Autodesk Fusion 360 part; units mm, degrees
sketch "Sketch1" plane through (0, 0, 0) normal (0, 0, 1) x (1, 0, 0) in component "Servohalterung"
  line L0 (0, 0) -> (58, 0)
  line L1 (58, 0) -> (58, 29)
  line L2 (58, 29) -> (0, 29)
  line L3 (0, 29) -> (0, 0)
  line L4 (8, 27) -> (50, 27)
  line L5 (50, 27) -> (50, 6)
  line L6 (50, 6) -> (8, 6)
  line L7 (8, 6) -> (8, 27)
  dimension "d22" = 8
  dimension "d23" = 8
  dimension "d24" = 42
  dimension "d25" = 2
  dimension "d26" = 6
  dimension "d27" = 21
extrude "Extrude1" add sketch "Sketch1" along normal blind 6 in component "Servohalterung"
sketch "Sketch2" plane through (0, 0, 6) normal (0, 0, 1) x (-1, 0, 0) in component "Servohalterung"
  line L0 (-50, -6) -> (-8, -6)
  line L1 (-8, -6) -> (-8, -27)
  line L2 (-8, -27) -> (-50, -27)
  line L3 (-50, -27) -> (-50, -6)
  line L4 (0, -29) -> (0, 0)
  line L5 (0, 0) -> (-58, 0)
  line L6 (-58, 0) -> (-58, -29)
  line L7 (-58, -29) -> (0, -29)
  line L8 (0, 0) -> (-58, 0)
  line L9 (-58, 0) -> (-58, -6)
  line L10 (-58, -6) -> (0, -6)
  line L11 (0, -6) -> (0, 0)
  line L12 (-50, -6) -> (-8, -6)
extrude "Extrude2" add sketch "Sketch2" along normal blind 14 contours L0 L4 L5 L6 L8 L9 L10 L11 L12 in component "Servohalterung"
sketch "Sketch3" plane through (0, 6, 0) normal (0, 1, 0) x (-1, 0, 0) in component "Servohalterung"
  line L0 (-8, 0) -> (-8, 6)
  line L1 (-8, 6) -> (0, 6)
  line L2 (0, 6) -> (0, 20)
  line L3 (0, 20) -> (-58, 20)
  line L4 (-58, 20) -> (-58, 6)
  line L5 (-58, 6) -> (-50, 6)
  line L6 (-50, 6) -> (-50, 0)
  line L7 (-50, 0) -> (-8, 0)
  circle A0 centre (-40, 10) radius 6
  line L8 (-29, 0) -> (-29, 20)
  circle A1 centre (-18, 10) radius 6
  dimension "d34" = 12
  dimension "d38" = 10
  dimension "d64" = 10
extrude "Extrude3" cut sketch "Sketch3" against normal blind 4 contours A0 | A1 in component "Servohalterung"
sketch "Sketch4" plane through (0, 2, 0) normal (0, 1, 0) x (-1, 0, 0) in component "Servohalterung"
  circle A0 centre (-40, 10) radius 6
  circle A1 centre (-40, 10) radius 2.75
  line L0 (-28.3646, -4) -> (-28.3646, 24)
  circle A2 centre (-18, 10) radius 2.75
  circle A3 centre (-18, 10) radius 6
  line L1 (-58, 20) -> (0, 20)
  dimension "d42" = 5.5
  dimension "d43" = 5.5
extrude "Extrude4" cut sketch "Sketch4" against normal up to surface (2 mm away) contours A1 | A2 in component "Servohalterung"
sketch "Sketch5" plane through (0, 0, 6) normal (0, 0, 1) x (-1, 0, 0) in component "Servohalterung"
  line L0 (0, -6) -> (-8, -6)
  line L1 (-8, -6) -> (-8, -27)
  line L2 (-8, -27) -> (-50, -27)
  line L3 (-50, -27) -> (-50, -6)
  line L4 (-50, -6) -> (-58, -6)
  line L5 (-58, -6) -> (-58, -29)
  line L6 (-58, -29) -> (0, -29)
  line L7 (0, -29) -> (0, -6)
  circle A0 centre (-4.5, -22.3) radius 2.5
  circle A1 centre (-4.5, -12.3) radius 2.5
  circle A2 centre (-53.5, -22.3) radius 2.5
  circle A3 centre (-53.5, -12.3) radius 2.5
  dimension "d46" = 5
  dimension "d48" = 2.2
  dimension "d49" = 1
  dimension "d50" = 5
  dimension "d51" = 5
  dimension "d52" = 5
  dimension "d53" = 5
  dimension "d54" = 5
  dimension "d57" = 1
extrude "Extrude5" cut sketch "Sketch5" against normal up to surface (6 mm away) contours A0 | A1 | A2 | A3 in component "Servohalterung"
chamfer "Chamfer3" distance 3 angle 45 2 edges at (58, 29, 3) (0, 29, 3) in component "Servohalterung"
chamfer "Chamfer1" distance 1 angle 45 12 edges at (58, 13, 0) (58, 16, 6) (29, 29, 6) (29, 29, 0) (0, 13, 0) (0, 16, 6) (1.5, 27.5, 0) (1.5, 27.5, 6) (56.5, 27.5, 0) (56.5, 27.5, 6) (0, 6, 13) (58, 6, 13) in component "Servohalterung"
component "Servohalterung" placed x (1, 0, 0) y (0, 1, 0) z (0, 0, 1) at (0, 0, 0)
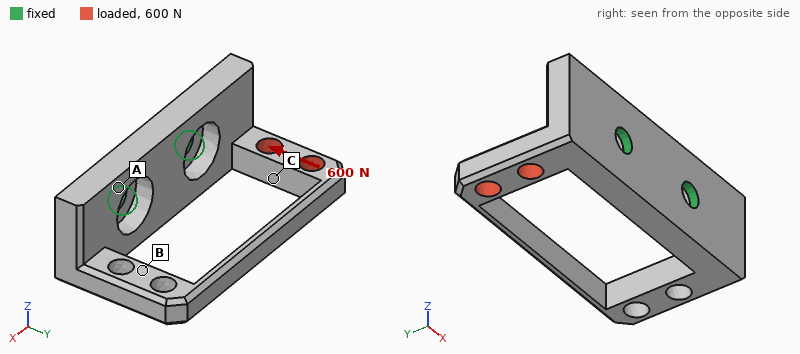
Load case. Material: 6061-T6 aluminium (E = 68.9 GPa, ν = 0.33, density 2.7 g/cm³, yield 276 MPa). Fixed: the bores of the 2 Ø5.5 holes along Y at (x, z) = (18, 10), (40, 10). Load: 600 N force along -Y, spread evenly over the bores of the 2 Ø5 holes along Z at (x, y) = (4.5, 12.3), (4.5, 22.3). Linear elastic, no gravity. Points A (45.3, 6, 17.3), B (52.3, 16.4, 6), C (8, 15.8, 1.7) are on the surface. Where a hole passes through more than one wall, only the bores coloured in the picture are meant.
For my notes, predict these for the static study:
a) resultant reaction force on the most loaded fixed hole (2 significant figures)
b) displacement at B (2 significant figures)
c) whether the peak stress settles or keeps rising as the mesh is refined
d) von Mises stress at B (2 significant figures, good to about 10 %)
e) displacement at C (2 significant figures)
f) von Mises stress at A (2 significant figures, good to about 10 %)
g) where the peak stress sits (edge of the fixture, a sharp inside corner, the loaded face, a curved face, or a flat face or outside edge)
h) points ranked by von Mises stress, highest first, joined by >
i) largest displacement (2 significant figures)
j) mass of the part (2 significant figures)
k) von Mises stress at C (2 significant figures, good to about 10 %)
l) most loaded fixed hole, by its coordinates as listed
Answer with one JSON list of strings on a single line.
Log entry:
["900 N", "0.035 mm", "keeps rising", "12 MPa", "0.093 mm", "22 MPa", "edge of the fixture", "C > A > B", "0.14 mm", "22 g", "42 MPa", "(18, 10)"]
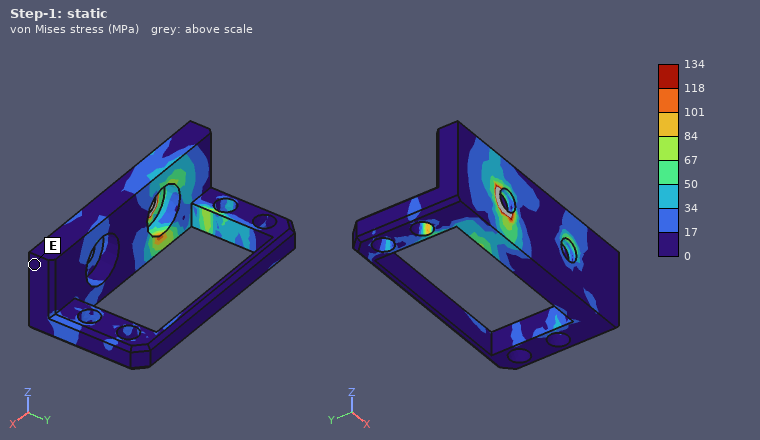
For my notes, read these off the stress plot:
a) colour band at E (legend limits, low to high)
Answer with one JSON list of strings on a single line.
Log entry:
["0 to 17 MPa"]
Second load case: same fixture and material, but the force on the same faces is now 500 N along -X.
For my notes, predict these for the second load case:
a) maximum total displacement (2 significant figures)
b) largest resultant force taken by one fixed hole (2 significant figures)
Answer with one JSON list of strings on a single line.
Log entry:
["0.15 mm", "410 N"]
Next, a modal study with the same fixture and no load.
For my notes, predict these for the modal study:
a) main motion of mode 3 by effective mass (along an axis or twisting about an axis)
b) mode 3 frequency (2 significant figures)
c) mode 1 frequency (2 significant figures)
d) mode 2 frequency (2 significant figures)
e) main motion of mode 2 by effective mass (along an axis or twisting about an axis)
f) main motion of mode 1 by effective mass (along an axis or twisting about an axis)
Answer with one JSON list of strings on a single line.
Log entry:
["twisting about Y", "4700 Hz", "3000 Hz", "3700 Hz", "along X", "along Z"]
